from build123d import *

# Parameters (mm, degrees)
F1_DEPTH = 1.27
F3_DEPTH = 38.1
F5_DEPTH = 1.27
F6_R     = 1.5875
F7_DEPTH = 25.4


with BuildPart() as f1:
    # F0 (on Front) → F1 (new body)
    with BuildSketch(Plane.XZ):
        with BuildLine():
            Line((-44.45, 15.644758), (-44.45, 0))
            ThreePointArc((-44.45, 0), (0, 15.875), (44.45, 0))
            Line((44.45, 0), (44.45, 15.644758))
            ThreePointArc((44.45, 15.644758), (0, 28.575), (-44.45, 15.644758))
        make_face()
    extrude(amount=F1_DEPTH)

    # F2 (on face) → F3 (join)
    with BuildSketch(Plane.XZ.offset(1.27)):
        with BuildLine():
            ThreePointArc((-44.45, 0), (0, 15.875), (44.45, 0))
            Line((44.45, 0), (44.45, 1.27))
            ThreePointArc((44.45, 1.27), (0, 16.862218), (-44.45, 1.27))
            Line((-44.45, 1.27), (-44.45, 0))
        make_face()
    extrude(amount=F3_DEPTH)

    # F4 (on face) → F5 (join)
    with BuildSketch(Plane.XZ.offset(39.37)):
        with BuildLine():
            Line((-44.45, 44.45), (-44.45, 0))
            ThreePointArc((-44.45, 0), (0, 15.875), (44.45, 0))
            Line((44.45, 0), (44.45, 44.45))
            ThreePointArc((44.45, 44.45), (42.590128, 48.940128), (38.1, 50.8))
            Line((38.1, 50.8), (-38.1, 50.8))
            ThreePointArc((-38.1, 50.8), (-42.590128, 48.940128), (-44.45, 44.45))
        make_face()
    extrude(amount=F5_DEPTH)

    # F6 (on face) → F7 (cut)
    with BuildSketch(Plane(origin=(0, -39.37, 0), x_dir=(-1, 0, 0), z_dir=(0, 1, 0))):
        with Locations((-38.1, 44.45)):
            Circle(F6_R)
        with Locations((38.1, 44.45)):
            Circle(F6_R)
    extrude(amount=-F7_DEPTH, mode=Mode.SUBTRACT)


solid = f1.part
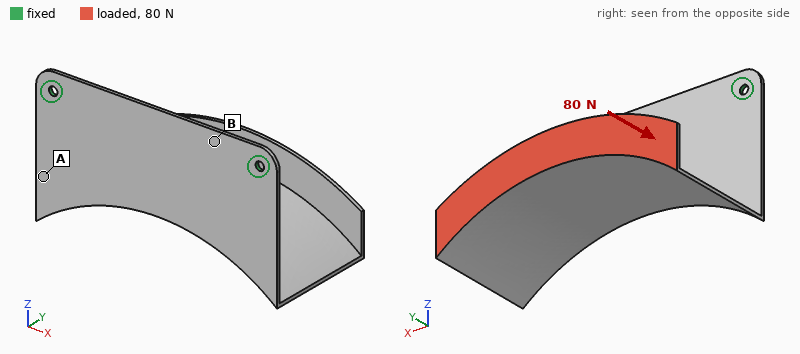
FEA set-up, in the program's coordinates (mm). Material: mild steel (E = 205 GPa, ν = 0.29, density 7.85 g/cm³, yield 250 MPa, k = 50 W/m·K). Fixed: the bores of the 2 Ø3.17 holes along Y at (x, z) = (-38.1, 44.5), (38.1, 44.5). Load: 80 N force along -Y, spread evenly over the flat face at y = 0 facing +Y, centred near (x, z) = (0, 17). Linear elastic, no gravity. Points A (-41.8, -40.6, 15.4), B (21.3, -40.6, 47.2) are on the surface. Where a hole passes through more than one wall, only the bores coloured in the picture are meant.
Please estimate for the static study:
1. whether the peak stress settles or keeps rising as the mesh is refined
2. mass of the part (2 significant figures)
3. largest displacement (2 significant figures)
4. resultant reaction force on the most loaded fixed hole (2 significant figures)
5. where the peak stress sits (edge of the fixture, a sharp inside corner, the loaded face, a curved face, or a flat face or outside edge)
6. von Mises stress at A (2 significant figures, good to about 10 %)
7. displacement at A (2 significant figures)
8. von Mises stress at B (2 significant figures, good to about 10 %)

keeps rising
75 g
0.80 mm
42 N
edge of the fixture
16 MPa
0.34 mm
55 MPa
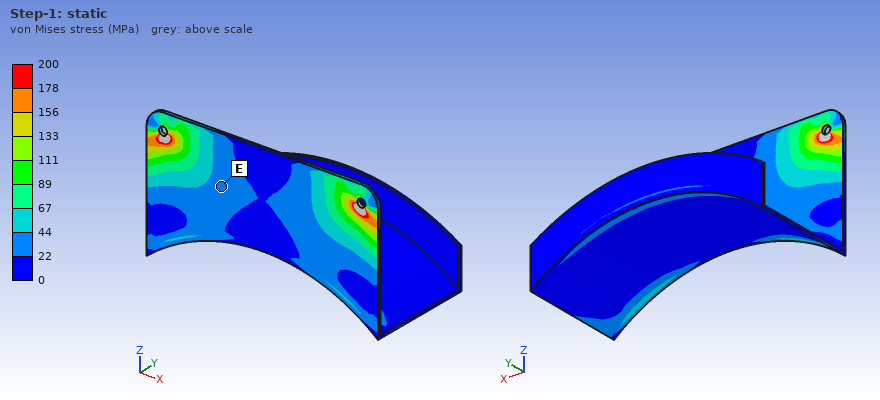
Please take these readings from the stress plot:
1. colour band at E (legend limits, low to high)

22 to 44 MPa
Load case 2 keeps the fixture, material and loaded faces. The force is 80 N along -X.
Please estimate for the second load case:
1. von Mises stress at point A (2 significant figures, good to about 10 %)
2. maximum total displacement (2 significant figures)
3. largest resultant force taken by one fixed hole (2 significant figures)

32 MPa
0.58 mm
66 N
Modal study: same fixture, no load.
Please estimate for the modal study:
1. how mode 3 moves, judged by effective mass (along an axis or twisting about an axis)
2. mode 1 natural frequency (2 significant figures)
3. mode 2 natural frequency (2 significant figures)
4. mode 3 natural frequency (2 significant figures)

along Y
190 Hz
340 Hz
530 Hz
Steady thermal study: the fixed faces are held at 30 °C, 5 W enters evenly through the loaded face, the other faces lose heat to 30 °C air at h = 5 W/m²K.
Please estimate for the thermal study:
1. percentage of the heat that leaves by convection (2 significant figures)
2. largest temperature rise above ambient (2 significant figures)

50 %
62 K
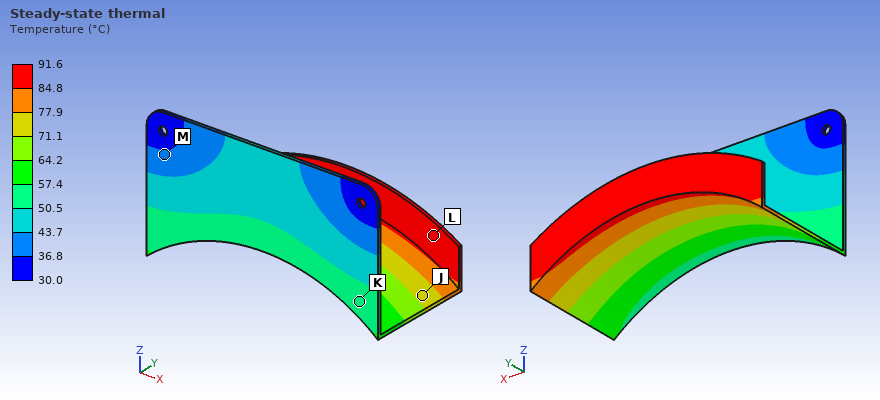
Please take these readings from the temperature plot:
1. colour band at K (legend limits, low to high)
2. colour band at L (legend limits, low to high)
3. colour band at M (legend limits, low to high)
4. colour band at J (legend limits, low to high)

50.5 to 57.4 °C
84.8 to 91.6 °C
36.8 to 43.7 °C
71.1 to 77.9 °C
